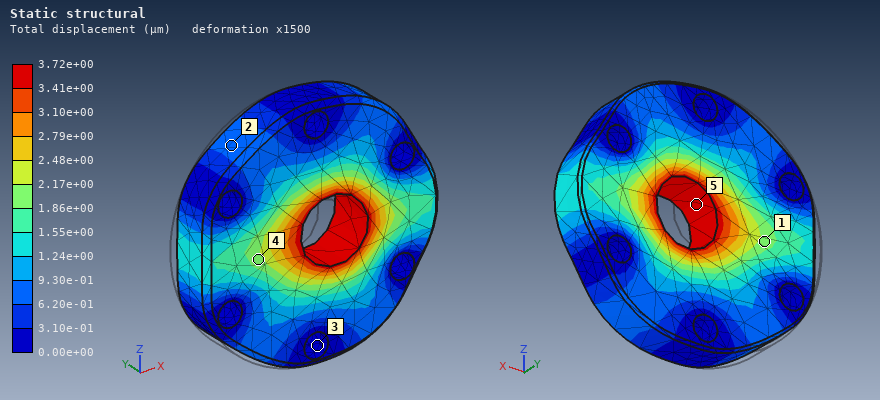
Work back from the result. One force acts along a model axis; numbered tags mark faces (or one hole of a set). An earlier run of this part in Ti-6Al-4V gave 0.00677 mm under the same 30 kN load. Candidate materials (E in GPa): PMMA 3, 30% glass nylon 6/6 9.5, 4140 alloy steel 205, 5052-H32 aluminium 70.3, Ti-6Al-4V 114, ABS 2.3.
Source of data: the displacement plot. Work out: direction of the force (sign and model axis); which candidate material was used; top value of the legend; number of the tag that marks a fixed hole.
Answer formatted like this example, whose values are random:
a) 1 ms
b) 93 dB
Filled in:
a) +X
b) 4140 alloy steel
c) 3.72e+00 µm
d) 3
